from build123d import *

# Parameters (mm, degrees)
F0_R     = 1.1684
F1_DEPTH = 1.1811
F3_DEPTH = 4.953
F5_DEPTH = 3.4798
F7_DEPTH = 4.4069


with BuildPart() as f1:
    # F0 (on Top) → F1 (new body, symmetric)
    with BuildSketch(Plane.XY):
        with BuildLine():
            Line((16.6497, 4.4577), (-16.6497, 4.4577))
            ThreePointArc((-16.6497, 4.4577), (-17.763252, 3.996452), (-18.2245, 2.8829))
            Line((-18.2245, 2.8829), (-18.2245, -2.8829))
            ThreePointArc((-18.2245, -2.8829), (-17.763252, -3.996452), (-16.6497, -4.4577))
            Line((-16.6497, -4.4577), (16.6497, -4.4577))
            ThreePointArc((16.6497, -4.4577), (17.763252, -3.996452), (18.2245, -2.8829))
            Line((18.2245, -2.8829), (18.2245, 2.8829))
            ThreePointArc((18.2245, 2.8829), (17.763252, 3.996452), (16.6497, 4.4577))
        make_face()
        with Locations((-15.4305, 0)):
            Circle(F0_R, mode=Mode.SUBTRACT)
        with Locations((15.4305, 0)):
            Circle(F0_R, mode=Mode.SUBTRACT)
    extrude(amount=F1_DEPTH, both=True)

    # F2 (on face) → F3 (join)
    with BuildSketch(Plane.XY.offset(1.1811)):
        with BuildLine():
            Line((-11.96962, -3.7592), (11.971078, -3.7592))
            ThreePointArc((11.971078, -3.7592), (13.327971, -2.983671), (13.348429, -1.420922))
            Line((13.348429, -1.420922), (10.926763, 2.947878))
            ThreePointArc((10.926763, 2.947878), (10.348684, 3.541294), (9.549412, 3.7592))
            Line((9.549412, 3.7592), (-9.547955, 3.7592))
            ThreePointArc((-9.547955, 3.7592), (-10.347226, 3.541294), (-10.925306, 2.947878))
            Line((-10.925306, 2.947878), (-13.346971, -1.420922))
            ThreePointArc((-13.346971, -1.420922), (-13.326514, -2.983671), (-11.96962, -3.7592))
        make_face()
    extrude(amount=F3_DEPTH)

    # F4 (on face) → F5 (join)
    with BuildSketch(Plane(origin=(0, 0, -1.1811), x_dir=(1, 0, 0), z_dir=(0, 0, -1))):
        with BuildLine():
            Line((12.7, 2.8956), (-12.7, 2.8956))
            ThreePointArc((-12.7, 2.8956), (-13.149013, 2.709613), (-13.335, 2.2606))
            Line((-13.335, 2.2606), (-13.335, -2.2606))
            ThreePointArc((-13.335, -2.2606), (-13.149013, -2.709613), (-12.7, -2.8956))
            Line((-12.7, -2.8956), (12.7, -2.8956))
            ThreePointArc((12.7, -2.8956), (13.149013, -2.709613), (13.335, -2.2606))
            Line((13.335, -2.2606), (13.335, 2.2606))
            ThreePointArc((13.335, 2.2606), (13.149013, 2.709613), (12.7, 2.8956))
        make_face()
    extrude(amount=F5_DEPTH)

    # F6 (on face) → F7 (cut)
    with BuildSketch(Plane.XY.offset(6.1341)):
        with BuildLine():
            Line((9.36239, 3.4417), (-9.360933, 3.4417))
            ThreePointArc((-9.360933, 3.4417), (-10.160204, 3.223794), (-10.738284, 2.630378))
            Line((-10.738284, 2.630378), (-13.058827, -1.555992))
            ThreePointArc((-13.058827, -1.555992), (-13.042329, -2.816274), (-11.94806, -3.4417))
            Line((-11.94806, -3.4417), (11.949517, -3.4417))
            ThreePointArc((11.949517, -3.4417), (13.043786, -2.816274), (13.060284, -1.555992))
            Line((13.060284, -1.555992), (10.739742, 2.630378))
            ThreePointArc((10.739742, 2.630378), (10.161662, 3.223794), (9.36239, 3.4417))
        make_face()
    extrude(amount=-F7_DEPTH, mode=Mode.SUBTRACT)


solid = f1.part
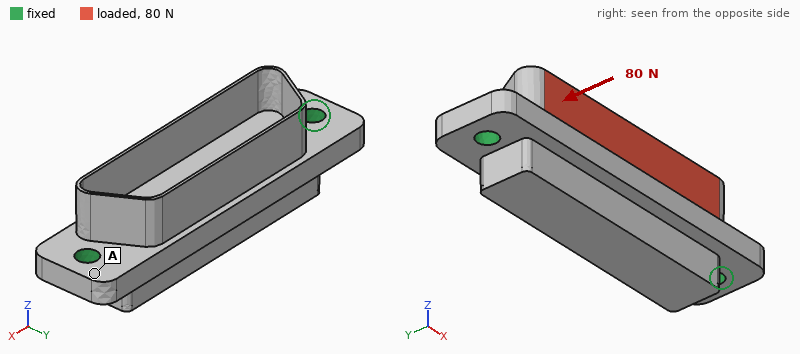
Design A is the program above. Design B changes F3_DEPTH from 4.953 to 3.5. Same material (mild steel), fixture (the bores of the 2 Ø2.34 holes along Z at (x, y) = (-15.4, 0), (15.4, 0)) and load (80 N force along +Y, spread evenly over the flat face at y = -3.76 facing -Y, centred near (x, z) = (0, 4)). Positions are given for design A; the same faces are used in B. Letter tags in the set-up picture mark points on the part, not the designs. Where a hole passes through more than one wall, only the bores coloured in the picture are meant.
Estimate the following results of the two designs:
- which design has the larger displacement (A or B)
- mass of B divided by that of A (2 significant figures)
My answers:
A
0.98
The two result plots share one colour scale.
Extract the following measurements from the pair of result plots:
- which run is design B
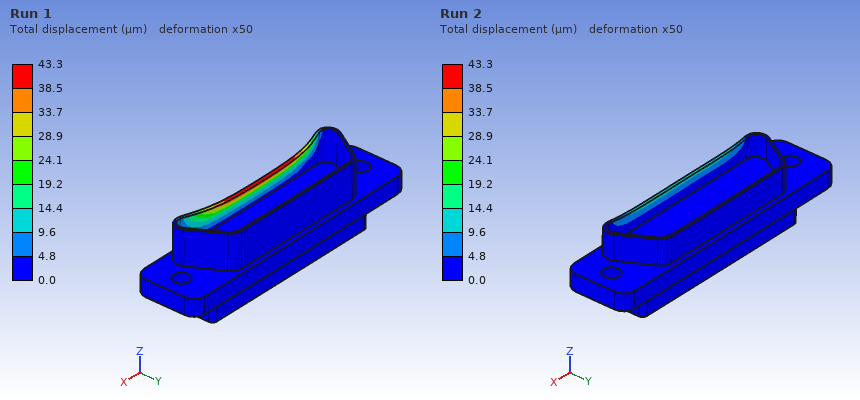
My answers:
Run 2
